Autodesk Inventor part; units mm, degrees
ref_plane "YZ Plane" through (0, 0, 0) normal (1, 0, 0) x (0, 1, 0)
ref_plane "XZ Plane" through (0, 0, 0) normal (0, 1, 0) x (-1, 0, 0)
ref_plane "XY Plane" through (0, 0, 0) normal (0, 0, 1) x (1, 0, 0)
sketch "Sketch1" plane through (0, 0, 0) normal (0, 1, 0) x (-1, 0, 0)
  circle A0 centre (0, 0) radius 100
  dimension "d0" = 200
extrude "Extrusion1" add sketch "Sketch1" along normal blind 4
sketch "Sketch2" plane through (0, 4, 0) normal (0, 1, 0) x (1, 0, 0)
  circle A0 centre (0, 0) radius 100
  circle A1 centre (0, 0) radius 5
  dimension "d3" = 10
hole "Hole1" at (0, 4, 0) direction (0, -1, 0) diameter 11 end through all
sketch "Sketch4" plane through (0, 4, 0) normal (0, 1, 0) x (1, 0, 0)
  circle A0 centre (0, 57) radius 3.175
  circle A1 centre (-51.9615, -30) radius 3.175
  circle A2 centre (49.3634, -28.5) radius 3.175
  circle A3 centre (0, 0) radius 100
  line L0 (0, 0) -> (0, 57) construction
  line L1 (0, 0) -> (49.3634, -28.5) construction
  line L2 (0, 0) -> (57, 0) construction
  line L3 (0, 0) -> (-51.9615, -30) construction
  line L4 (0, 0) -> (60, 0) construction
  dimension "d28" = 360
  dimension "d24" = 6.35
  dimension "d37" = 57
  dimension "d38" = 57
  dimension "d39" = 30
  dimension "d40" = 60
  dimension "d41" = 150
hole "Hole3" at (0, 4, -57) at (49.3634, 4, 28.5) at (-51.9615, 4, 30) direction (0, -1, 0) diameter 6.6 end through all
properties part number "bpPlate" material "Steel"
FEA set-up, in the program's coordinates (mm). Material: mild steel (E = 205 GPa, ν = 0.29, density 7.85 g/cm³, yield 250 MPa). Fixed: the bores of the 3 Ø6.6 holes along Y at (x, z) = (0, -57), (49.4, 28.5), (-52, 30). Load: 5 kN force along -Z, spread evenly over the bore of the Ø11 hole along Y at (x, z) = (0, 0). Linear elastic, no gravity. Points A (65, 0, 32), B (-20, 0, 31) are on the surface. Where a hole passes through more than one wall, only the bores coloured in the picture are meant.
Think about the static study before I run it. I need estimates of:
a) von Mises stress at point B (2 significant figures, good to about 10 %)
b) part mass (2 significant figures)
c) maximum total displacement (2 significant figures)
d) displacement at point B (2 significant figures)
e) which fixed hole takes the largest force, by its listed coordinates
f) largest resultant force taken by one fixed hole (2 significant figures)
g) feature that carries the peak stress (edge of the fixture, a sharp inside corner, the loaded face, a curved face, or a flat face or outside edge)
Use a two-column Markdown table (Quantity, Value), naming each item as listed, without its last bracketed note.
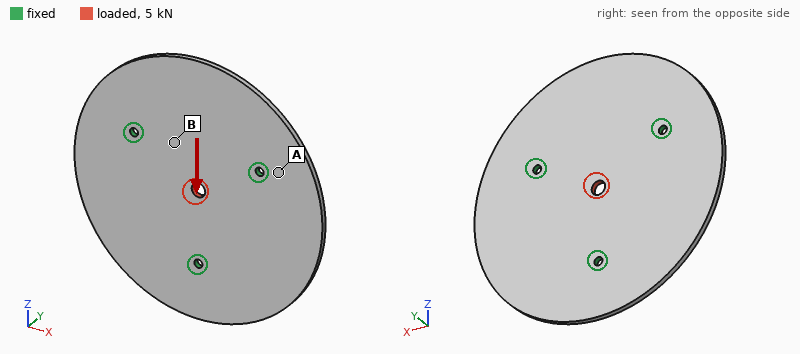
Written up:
| Quantity | Value |
|---|---|
| von Mises stress at point B | 7.6 MPa |
| part mass | 980 g |
| maximum total displacement | 5.3 µm |
| displacement at point B | 2.4 µm |
| which fixed hole takes the largest force, by its listed coordinates | (0, -57) |
| largest resultant force taken by one fixed hole | 1.9 kN |
| feature that carries the peak stress | the loaded face |
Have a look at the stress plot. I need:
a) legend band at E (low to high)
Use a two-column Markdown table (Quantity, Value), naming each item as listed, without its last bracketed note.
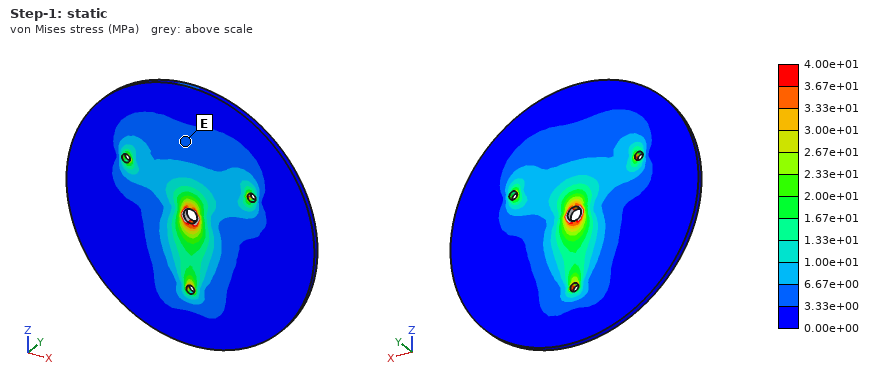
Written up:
| Quantity | Value |
|---|---|
| legend band at E | 3.33e+00 to 6.67e+00 MPa |
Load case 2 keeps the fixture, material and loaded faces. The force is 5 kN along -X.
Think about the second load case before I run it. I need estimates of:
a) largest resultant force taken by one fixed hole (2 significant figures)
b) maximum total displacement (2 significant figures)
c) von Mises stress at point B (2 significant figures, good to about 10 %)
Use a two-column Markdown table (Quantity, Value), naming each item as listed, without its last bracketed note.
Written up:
| Quantity | Value |
|---|---|
| largest resultant force taken by one fixed hole | 1.8 kN |
| maximum total displacement | 5.3 µm |
| von Mises stress at point B | 6.5 MPa |
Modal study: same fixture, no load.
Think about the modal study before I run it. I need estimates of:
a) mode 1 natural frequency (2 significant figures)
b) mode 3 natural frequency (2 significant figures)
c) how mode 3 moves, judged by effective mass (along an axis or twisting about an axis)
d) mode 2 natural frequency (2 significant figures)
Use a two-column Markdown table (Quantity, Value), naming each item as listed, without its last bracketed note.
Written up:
| Quantity | Value |
|---|---|
| mode 1 natural frequency | 670 Hz |
| mode 3 natural frequency | 810 Hz |
| how mode 3 moves, judged by effective mass | along Y |
| mode 2 natural frequency | 680 Hz |
